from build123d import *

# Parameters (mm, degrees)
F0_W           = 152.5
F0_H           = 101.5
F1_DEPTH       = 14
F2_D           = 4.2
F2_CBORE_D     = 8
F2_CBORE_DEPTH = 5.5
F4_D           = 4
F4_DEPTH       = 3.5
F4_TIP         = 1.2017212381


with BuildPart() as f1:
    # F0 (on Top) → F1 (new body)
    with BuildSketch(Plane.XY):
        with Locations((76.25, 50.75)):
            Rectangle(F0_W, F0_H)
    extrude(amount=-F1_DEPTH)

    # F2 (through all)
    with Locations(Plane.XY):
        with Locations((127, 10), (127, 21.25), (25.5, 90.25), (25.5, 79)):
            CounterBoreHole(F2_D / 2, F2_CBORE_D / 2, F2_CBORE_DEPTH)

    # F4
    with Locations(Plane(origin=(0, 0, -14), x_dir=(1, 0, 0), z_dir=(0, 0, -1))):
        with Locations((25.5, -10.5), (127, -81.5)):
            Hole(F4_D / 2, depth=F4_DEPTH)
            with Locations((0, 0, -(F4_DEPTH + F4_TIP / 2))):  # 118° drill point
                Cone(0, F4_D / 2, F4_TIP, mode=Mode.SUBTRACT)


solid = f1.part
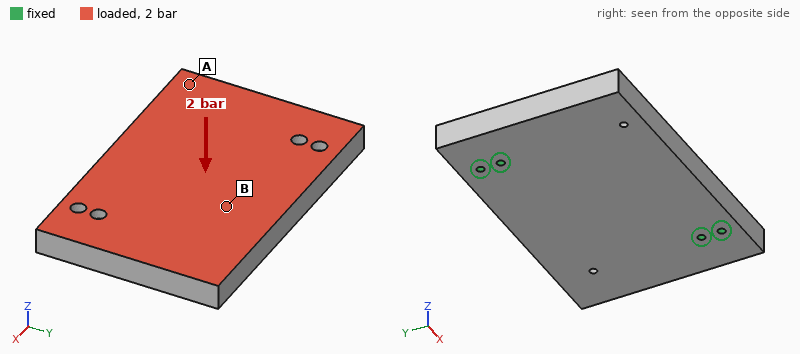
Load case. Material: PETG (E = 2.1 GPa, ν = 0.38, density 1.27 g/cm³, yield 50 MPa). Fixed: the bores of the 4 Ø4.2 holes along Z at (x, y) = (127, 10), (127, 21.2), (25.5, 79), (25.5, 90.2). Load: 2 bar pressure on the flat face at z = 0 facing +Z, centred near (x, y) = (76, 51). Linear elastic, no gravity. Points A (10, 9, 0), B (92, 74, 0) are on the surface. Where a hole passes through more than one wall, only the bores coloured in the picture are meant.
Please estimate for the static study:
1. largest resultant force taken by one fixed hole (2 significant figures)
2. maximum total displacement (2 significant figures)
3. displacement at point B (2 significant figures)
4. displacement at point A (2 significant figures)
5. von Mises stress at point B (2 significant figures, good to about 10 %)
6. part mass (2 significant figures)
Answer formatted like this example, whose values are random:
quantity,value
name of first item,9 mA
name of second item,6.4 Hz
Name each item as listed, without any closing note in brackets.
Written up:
quantity,value
largest resultant force taken by one fixed hole,1.8 kN
maximum total displacement,1.9 mm
displacement at point B,0.94 mm
displacement at point A,1.5 mm
von Mises stress at point B,8.2 MPa
part mass,270 g
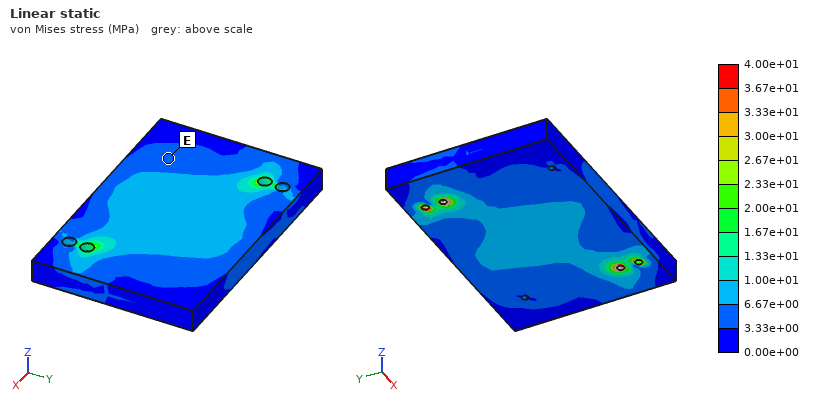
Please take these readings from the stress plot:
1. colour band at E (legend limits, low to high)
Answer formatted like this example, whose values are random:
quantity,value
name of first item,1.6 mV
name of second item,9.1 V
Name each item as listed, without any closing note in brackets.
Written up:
quantity,value
colour band at E,3.33e+00 to 6.67e+00 MPa
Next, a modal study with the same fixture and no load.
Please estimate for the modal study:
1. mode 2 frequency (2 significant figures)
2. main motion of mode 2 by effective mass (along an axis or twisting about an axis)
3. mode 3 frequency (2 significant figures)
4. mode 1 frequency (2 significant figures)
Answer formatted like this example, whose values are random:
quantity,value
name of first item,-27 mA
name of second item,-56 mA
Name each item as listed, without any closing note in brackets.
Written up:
quantity,value
mode 2 frequency,530 Hz
main motion of mode 2 by effective mass,along Z
mode 3 frequency,990 Hz
mode 1 frequency,370 Hz
